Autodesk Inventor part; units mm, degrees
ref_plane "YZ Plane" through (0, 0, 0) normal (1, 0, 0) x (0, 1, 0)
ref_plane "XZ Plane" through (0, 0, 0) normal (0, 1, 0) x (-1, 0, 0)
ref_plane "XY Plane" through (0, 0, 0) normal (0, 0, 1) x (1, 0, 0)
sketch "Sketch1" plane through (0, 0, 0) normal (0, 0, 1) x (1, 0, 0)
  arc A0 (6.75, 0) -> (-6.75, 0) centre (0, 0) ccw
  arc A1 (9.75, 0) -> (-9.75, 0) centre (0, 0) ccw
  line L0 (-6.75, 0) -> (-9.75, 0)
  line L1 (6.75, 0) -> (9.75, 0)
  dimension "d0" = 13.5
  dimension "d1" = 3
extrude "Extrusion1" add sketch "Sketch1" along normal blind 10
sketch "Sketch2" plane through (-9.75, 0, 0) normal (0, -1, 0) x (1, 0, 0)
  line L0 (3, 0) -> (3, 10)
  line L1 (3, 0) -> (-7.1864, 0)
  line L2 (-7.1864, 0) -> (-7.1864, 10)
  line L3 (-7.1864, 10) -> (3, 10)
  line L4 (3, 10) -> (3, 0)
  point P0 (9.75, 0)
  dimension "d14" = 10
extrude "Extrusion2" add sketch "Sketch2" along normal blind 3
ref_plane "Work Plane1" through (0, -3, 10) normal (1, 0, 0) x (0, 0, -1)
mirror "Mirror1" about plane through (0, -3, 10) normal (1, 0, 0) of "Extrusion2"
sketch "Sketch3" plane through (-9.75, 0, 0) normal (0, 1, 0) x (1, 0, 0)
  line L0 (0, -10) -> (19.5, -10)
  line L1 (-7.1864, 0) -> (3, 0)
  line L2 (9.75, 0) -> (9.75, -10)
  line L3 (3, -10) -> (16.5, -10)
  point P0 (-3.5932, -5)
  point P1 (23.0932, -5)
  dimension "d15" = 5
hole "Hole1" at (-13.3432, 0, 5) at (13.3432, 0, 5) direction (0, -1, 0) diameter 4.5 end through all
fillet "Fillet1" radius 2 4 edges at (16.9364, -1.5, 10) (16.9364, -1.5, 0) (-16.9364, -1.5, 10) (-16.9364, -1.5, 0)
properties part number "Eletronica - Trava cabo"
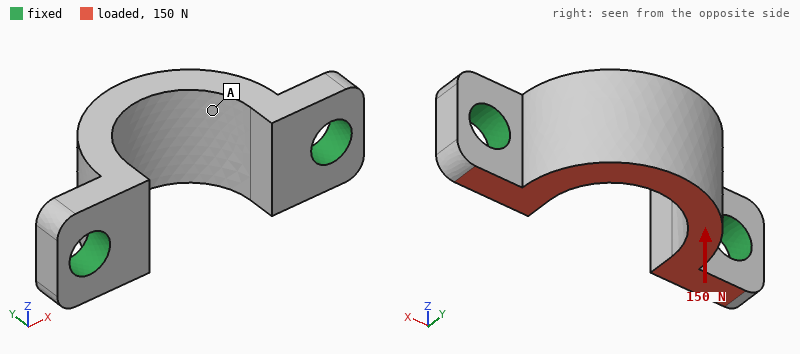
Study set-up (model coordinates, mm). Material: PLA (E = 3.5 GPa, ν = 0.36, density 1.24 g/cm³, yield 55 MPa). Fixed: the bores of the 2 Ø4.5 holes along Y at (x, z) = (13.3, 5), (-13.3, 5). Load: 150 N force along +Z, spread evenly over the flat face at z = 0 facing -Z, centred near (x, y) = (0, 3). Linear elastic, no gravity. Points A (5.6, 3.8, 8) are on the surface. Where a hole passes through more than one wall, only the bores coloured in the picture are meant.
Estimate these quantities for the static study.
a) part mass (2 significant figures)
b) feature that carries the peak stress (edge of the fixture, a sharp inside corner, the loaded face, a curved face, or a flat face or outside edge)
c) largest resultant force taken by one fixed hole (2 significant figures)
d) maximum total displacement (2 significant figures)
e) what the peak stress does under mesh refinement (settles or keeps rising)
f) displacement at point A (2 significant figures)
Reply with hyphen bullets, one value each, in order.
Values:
- 1.6 g
- edge of the fixture
- 75 N
- 0.12 mm
- keeps rising
- 0.058 mm
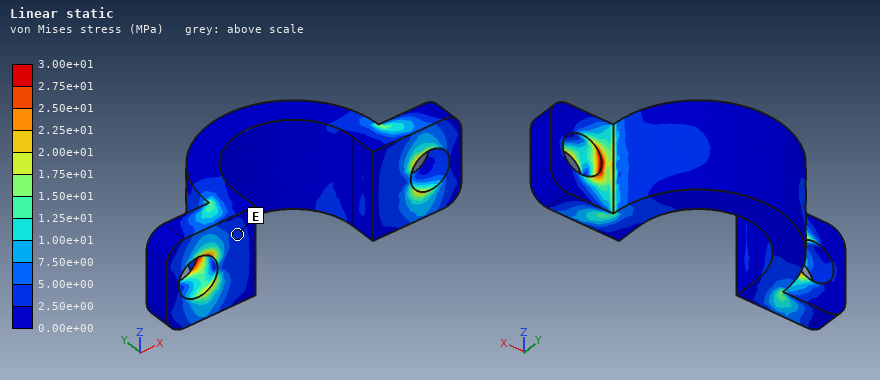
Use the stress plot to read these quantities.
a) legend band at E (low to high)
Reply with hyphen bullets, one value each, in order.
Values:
- 2.50e+00 to 5.00e+00 MPa
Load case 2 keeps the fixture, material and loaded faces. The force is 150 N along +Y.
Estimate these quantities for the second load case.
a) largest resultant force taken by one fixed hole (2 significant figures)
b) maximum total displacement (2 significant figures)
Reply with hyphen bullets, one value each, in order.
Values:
- 79 N
- 0.11 mm
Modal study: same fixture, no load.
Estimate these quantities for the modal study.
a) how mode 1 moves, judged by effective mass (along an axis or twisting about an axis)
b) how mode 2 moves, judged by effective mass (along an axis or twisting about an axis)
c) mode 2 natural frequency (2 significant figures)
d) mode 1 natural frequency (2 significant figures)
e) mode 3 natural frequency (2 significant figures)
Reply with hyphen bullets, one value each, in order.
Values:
- along Z
- along X
- 8600 Hz
- 5400 Hz
- 12 kHz
